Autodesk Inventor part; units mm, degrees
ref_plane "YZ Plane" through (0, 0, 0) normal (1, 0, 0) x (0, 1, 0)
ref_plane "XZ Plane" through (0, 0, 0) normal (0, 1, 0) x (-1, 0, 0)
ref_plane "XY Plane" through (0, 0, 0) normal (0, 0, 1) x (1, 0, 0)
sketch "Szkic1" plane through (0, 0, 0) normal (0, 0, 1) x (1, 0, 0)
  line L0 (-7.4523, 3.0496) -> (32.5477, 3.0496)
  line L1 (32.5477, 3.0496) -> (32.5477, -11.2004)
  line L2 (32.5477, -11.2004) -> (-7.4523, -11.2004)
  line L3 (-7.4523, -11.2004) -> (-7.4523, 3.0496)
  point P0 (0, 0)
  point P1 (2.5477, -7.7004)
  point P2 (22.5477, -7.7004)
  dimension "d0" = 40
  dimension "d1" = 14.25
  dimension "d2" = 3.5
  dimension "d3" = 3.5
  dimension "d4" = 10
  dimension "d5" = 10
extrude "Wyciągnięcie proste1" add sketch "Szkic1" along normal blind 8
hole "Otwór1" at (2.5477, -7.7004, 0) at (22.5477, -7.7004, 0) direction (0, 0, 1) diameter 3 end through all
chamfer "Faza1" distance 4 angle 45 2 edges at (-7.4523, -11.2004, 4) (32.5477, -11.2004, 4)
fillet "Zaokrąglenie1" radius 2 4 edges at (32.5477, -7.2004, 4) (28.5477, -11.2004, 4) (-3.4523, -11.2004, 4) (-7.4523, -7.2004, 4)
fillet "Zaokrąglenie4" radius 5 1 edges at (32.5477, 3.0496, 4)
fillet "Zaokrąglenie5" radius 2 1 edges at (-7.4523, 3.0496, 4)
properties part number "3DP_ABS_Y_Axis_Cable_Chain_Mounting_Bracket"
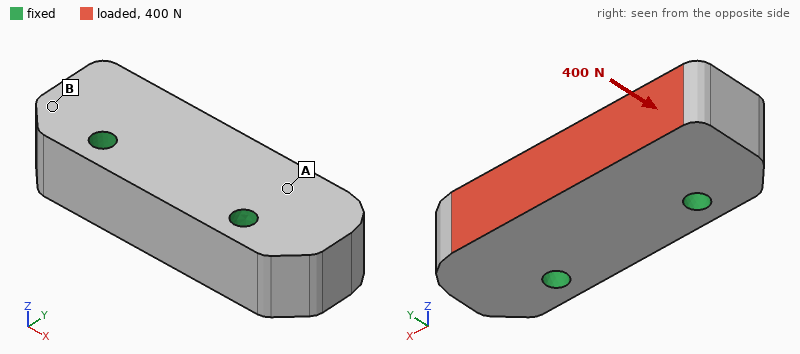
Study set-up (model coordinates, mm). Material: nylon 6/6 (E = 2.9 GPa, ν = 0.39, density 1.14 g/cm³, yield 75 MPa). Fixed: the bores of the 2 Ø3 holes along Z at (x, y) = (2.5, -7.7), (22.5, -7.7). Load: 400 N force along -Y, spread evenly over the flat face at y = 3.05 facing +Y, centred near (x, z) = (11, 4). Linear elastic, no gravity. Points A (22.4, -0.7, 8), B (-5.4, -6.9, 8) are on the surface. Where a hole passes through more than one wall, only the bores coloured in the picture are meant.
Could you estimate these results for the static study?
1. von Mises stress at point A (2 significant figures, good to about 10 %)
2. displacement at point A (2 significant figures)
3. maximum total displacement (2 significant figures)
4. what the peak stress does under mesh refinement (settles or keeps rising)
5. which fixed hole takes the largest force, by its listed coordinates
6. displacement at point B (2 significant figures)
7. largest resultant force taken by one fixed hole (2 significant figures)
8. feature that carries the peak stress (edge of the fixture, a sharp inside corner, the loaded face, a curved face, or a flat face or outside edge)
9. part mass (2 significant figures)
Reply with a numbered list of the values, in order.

1. 1.9 MPa
2. 4.9 µm
3. 12 µm
4. keeps rising
5. (2.5, -7.7)
6. 8.7 µm
7. 230 N
8. edge of the fixture
9. 4.9 g
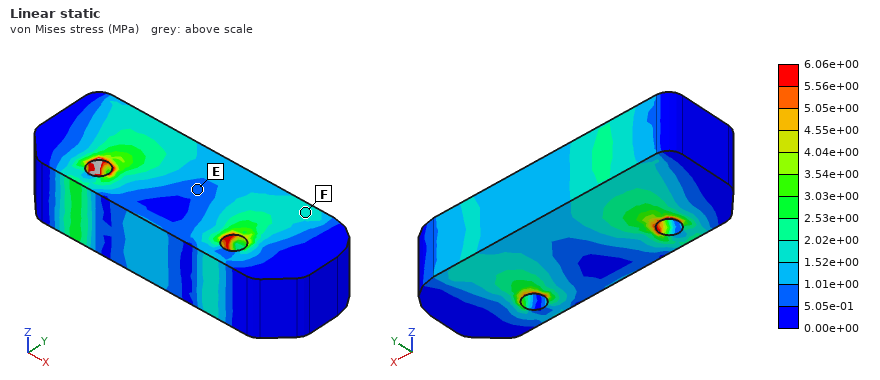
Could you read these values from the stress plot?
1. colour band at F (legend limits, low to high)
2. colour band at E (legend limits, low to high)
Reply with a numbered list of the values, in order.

1. 1.52e+00 to 2.02e+00 MPa
2. 5.05e-01 to 1.01e+00 MPa
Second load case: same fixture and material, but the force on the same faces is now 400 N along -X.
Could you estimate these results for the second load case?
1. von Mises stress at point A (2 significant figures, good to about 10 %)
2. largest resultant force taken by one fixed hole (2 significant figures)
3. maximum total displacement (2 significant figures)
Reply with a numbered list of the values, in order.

1. 2.2 MPa
2. 270 N
3. 43 µm
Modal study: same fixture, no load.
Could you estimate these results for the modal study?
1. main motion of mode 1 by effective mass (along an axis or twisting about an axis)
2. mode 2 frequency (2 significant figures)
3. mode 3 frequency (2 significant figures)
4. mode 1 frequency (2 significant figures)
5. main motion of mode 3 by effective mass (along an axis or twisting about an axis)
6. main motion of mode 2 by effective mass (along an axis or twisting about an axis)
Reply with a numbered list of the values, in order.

1. along Z
2. 11 kHz
3. 12 kHz
4. 9800 Hz
5. along X
6. twisting about Y
